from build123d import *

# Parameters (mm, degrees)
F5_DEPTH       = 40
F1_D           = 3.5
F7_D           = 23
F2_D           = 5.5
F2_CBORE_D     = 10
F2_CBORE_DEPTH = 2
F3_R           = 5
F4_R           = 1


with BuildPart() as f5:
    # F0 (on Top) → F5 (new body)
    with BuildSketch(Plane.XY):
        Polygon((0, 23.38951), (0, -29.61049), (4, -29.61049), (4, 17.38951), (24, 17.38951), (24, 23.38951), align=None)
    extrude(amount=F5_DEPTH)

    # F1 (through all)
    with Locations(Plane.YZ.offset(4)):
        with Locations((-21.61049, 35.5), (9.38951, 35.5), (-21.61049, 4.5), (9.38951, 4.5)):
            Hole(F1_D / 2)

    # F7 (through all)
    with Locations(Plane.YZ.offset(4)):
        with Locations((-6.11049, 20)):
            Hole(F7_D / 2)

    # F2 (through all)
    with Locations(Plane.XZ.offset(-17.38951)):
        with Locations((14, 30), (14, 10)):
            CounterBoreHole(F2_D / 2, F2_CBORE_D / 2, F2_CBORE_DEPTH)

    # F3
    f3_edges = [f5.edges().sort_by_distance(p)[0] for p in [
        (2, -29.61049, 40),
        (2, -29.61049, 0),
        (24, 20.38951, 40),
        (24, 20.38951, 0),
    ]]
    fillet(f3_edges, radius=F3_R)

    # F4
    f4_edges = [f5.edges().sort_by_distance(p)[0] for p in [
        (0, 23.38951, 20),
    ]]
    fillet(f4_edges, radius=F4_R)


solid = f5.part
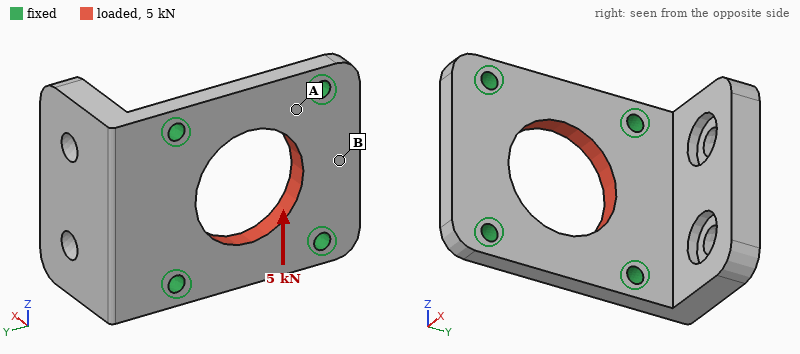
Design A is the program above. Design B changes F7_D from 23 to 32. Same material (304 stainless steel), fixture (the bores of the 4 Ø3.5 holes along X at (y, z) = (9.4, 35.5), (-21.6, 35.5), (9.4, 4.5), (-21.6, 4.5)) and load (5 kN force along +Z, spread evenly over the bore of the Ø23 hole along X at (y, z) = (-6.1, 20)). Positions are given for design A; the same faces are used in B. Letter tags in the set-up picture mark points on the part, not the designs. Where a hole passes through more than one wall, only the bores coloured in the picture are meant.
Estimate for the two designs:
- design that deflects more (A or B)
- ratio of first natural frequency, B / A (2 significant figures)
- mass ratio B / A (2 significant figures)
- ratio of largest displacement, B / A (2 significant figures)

B
0.95
0.86
1.9
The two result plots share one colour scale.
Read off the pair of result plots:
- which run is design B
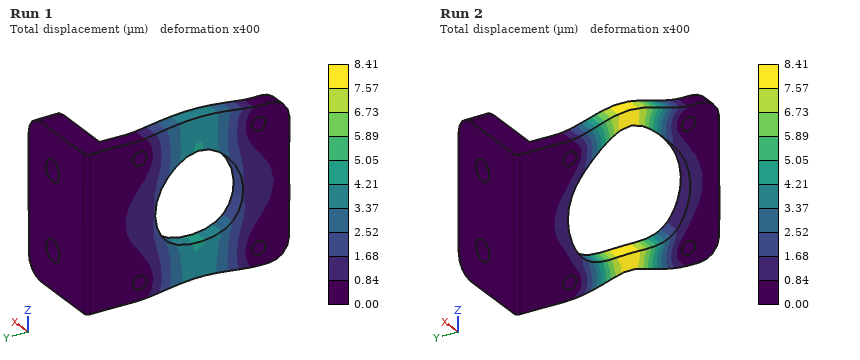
Run 2
